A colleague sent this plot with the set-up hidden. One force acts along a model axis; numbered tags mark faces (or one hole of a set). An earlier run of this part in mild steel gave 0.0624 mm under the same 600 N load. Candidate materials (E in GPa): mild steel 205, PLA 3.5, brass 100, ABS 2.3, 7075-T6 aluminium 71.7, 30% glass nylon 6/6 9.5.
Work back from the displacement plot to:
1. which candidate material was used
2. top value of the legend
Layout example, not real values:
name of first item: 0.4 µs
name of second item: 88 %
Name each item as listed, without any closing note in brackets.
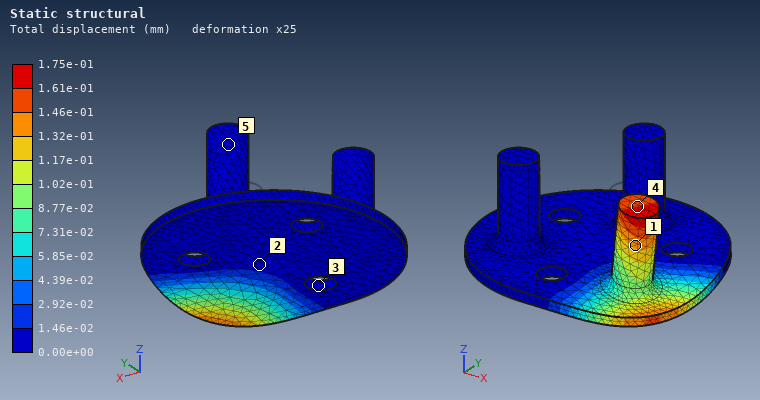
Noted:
which candidate material was used: 7075-T6 aluminium
top value of the legend: 1.75e-01 mm
